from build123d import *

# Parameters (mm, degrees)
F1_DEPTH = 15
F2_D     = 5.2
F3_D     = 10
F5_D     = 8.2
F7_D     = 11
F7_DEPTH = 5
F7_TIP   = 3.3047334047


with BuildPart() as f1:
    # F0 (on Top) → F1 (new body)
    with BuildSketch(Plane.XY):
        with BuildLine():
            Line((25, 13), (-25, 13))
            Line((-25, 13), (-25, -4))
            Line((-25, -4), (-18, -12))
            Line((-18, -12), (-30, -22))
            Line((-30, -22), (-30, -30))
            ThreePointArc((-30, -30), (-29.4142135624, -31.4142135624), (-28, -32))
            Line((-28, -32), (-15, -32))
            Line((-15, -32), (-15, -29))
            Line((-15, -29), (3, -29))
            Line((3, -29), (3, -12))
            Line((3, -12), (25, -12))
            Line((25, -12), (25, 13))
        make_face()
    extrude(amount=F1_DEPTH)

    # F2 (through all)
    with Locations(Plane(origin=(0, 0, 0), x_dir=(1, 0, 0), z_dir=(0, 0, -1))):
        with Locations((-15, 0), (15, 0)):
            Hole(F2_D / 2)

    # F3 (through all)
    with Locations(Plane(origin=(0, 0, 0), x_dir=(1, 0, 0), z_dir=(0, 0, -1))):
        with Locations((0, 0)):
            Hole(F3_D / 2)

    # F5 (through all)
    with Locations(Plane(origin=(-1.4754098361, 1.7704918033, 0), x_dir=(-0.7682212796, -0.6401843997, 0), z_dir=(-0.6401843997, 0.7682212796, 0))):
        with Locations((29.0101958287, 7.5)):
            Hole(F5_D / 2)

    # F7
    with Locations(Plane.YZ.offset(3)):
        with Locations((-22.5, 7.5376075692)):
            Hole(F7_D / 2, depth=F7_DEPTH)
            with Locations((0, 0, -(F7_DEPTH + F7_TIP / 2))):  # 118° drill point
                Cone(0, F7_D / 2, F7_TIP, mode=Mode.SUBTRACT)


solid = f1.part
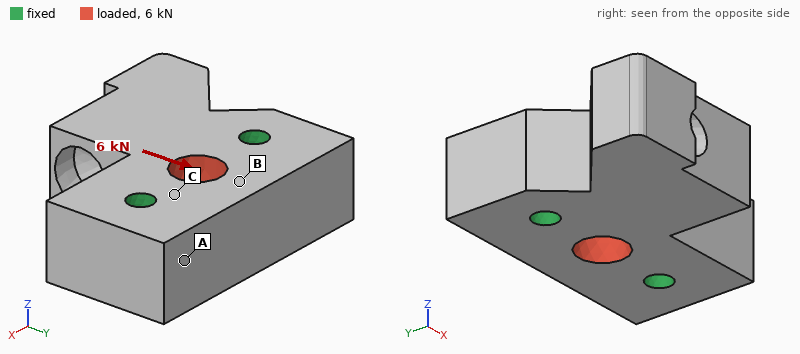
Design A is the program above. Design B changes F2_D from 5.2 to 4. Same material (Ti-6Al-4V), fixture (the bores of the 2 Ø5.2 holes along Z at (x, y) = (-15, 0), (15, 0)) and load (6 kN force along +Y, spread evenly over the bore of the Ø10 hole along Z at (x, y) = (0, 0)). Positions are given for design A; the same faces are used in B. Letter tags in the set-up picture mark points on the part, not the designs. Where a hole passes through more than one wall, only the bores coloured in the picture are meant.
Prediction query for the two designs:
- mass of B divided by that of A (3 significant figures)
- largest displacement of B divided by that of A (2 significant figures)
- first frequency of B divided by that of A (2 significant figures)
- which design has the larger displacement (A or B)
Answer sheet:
1.01
1.1
0.96
B
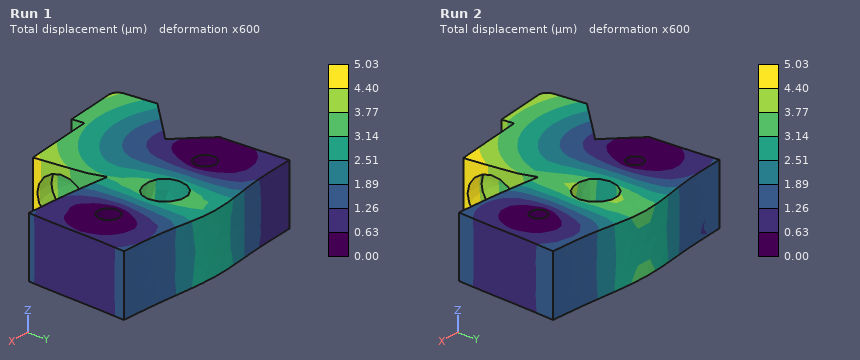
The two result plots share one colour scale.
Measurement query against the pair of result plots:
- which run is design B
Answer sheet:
Run 2
